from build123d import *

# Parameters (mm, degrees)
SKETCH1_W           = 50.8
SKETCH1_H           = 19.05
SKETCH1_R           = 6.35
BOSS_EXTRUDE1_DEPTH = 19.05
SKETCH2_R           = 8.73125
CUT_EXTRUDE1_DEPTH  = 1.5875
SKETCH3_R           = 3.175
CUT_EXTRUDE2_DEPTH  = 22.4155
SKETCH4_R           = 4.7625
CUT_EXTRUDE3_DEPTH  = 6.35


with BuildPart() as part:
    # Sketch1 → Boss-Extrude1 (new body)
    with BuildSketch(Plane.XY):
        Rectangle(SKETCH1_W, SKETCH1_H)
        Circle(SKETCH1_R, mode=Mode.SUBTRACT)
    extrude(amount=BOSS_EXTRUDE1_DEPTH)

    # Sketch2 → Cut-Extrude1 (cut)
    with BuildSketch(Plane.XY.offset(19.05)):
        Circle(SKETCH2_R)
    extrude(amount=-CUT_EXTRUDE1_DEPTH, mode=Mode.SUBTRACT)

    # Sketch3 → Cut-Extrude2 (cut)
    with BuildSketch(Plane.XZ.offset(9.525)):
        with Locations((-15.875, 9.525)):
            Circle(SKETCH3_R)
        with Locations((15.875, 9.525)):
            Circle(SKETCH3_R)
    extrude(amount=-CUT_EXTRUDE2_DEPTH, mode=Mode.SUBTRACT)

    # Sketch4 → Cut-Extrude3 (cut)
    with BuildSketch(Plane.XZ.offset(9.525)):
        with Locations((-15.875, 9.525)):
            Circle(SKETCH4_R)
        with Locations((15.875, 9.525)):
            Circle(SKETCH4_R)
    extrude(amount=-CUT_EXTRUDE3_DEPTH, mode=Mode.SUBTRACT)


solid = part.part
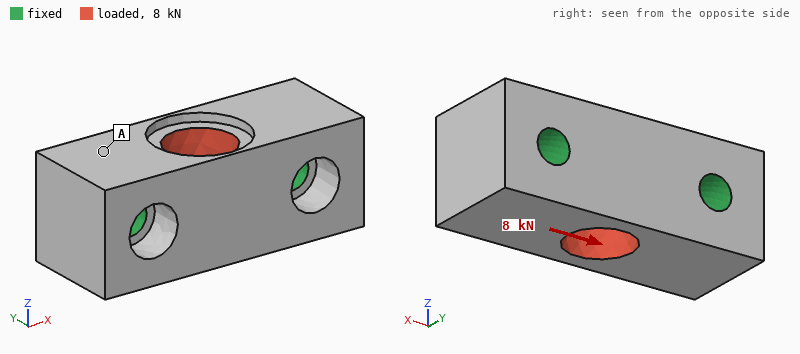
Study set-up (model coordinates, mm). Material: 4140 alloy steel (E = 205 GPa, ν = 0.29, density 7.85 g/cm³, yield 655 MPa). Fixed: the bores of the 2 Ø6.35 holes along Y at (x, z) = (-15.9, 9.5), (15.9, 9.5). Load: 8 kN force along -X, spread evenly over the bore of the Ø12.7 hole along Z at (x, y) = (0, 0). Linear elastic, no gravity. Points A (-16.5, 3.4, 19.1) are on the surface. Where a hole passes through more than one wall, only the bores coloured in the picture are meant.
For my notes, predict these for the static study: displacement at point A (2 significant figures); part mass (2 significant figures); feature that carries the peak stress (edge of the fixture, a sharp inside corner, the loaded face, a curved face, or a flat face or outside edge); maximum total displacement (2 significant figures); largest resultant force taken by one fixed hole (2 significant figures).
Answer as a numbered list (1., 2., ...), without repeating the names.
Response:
1. 0.35 µm
2. 110 g
3. edge of the fixture
4. 2.0 µm
5. 4.0 kN
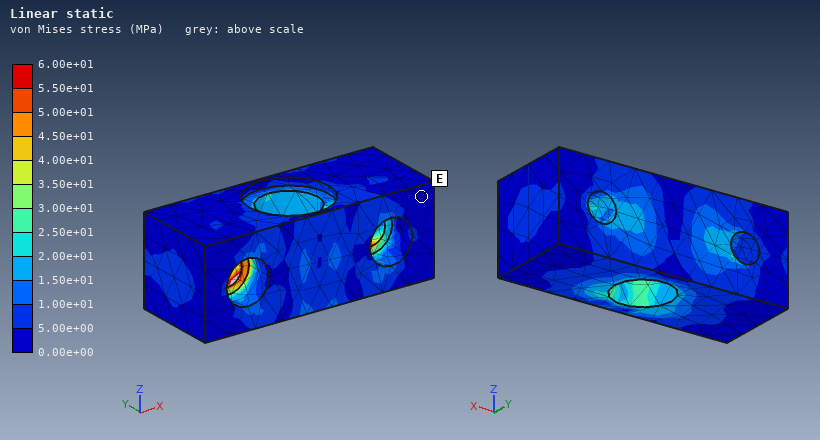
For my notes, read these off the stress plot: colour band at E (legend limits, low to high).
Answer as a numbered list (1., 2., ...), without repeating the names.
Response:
1. 0.00e+00 to 5.00e+00 MPa
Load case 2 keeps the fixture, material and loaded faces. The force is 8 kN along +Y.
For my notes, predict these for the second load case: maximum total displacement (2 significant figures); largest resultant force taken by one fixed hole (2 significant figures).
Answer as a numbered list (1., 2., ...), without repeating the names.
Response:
1. 4.3 µm
2. 4.0 kN
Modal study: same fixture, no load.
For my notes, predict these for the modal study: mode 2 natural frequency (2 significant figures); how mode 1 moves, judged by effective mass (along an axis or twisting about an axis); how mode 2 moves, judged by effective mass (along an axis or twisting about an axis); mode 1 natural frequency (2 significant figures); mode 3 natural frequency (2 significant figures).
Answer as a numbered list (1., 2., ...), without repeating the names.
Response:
1. 37 kHz
2. along Z
3. twisting about X
4. 31 kHz
5. 40 kHz
